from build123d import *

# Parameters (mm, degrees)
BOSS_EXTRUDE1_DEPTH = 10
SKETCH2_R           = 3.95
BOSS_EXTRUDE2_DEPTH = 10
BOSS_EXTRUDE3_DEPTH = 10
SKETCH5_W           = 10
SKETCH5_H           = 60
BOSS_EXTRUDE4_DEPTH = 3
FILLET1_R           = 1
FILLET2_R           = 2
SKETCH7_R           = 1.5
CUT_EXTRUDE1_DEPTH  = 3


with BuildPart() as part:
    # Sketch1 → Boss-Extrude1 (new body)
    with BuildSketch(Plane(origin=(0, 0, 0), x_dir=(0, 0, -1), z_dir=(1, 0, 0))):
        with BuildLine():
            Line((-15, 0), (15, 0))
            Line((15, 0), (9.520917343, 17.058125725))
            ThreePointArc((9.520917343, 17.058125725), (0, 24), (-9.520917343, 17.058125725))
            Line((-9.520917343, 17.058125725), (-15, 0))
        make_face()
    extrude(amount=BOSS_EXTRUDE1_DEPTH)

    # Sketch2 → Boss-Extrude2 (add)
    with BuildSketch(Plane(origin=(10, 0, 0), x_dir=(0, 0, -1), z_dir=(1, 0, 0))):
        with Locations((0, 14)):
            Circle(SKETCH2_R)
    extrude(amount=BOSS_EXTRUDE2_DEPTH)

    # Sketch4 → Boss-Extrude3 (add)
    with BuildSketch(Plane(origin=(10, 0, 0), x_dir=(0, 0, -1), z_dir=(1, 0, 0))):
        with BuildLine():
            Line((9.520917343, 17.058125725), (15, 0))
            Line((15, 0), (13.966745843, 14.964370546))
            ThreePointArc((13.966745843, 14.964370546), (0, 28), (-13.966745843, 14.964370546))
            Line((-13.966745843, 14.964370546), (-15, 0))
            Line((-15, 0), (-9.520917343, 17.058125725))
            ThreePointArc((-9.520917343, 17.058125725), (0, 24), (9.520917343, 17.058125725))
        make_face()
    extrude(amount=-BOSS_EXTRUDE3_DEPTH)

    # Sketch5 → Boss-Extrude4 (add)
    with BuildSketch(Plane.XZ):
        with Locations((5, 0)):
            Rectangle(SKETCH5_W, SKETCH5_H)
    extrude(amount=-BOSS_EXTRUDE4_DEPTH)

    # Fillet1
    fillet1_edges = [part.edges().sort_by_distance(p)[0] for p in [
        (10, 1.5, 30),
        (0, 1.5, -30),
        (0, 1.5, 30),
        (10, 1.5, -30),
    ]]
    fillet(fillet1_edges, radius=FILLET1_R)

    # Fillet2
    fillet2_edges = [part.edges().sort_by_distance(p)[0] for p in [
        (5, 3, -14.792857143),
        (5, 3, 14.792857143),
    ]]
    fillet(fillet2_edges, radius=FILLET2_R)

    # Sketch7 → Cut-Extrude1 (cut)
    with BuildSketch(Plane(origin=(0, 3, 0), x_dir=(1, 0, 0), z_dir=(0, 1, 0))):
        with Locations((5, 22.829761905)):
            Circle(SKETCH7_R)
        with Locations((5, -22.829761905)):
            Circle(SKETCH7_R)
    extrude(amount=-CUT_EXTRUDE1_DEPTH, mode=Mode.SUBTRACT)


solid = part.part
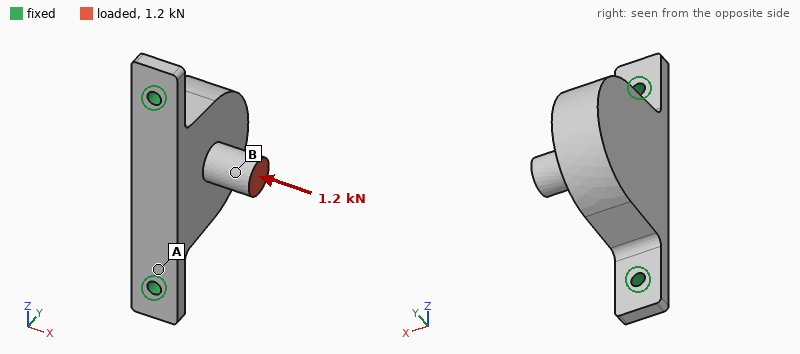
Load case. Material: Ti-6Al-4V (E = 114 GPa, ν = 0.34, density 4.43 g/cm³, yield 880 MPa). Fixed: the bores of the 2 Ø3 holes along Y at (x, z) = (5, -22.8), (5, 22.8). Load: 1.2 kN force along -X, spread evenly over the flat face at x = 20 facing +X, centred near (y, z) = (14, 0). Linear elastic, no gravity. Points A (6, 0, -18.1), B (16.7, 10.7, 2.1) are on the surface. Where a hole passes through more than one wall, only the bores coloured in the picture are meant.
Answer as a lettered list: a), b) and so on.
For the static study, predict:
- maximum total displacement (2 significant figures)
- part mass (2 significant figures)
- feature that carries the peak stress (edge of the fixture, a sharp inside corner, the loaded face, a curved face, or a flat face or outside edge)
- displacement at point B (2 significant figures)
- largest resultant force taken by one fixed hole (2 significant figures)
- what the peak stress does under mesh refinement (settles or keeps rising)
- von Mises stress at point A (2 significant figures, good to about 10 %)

a) 0.43 mm
b) 38 g
c) edge of the fixture
d) 0.24 mm
e) 600 N
f) keeps rising
g) 300 MPa
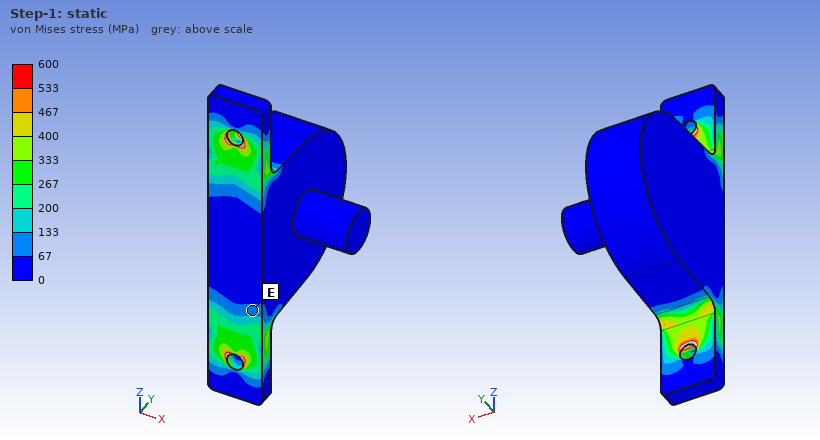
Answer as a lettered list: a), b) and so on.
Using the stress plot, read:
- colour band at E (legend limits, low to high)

a) 67 to 133 MPa
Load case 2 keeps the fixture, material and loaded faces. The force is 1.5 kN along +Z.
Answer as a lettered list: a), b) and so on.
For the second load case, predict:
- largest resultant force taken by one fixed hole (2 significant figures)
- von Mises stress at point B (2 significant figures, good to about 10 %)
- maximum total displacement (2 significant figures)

a) 1.1 kN
b) 77 MPa
c) 77 µm
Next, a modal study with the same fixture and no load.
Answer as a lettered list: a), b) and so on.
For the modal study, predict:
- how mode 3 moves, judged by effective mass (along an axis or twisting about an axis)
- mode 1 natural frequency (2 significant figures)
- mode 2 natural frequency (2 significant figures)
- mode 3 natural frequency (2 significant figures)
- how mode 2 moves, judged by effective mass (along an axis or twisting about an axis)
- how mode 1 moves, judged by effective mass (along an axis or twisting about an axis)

a) along Z
b) 1900 Hz
c) 7100 Hz
d) 8500 Hz
e) along Y
f) along X
